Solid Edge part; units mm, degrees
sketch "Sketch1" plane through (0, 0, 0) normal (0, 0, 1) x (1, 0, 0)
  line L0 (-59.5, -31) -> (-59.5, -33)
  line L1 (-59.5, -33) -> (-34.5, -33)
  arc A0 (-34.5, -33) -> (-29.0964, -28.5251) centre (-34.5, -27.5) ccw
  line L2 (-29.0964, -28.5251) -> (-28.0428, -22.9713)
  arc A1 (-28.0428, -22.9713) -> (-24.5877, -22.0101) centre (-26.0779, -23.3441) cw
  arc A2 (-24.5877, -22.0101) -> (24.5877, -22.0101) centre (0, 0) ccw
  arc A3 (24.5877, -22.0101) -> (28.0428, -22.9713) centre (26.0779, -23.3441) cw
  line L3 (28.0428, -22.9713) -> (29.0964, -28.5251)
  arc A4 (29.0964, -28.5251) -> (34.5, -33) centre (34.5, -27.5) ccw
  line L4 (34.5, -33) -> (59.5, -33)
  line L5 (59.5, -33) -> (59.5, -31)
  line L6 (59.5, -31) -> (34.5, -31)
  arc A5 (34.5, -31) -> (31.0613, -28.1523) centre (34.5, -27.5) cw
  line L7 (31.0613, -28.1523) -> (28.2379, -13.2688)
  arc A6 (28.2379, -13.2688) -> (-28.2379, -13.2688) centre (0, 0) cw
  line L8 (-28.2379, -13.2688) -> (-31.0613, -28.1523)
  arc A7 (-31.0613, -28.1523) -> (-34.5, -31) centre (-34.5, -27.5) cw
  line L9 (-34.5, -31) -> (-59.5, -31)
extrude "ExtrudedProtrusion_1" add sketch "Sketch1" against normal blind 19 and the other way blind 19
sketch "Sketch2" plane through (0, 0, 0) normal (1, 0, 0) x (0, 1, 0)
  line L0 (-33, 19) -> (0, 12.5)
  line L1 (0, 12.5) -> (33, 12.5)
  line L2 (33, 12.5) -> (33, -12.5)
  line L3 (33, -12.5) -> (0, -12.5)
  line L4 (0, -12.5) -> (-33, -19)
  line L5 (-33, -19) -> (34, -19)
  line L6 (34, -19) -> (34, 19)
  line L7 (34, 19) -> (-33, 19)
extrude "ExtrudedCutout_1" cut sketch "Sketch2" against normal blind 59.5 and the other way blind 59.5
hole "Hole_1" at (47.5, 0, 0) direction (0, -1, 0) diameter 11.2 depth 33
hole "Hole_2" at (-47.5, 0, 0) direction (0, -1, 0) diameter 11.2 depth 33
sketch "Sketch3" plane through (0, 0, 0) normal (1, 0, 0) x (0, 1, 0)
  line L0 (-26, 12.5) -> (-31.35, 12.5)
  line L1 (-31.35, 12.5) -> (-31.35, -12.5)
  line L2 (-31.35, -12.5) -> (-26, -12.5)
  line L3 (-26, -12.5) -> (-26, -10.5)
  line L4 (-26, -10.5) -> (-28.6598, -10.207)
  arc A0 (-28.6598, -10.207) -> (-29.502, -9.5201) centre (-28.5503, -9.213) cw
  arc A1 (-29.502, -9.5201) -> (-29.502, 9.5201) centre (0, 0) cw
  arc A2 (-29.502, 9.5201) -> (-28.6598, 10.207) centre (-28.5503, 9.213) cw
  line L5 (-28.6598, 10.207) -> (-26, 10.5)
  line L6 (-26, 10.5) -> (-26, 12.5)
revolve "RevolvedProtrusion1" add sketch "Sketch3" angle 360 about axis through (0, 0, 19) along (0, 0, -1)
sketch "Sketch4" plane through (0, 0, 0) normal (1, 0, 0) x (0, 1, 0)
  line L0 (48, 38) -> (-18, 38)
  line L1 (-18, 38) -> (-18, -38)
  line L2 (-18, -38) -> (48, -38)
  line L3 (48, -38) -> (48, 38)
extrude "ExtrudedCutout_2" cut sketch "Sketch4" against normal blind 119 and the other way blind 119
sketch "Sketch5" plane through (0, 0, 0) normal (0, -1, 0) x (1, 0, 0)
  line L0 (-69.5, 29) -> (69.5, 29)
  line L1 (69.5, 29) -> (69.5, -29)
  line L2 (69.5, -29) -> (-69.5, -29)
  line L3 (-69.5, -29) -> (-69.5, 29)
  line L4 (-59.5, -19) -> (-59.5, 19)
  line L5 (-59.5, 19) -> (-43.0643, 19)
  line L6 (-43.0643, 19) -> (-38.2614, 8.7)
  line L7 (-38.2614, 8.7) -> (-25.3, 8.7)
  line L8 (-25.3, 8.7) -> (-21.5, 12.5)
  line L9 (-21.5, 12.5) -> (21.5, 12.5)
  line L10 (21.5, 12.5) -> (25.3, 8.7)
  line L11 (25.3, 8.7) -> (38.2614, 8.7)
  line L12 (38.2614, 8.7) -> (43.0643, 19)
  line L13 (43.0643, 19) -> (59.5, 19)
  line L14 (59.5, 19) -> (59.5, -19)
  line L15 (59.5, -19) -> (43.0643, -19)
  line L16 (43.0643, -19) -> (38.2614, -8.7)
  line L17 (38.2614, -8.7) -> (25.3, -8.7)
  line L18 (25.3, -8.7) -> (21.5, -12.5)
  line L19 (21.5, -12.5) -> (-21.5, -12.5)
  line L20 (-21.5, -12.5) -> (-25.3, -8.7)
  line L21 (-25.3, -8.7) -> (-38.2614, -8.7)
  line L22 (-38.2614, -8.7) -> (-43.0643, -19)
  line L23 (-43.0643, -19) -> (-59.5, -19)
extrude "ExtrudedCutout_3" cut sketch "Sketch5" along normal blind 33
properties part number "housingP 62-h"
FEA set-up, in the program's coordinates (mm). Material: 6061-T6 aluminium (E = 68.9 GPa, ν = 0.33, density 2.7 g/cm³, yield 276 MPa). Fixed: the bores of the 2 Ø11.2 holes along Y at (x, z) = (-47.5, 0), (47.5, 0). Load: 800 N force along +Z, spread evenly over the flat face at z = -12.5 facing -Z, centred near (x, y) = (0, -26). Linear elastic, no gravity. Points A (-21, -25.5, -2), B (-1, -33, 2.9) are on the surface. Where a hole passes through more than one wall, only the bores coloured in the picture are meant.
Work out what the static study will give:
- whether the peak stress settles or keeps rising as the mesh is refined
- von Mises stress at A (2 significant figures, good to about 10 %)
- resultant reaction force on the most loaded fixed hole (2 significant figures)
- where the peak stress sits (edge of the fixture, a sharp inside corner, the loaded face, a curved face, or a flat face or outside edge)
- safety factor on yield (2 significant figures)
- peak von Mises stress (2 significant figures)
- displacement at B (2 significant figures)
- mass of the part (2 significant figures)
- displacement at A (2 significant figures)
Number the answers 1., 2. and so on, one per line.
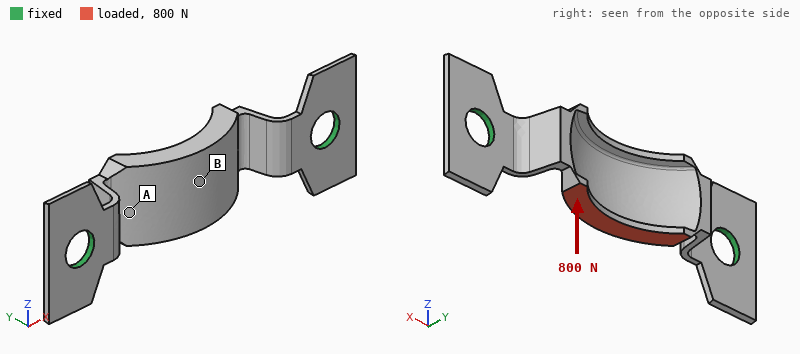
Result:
1. settles
2. 44 MPa
3. 400 N
4. a curved face
5. 1.8
6. 150 MPa
7. 0.098 mm
8. 24 g
9. 0.12 mm
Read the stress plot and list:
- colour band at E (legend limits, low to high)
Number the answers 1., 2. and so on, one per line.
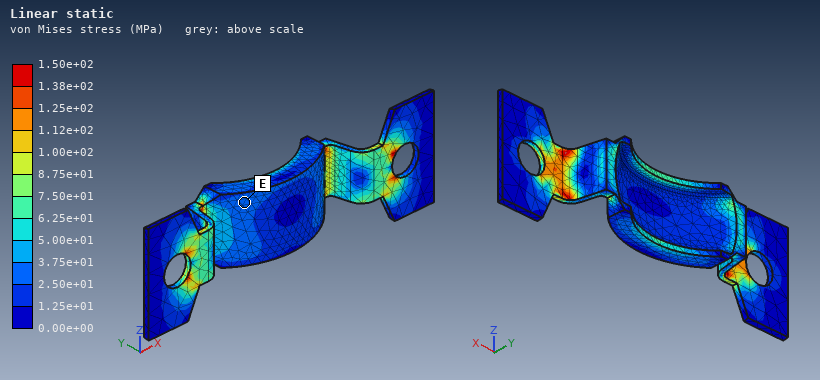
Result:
1. 2.50e+01 to 3.75e+01 MPa
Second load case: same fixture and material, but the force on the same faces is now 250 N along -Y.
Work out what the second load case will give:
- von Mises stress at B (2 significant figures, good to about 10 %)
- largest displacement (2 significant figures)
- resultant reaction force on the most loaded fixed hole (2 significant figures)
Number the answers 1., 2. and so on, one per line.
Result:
1. 16 MPa
2. 0.30 mm
3. 170 N
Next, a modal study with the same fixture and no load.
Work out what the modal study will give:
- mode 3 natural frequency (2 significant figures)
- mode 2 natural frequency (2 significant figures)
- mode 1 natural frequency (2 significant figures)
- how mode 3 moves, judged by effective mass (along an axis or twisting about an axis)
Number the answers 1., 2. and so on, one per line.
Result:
1. 2500 Hz
2. 2300 Hz
3. 2200 Hz
4. along X
